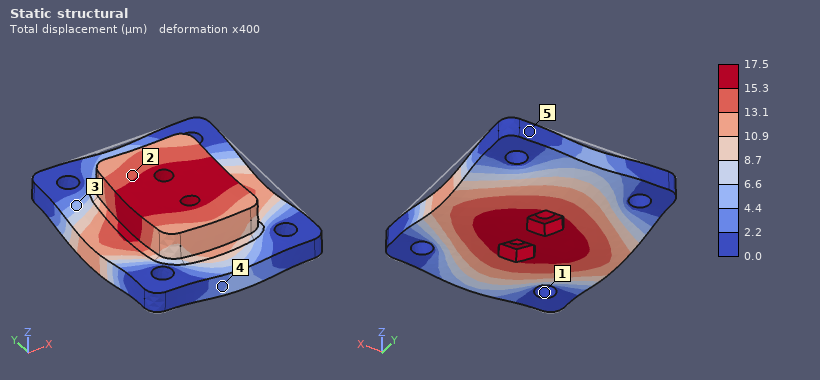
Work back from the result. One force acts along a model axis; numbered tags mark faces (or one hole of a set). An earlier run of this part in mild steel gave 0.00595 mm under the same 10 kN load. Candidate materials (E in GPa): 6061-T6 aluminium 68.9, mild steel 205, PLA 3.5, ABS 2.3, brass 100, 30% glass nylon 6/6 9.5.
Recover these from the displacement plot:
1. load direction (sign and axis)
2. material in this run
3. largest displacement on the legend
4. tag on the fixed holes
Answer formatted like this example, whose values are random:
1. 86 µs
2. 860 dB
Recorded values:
1. -Z
2. 6061-T6 aluminium
3. 17.5 µm
4. 1
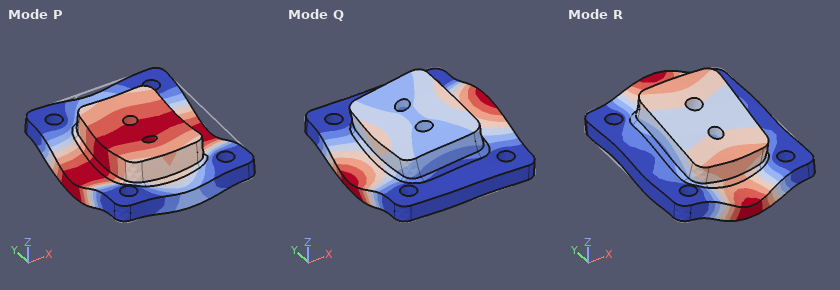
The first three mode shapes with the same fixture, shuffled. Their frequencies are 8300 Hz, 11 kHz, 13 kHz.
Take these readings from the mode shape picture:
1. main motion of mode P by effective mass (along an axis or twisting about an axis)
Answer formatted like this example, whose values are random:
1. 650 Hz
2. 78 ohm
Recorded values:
1. along Z
